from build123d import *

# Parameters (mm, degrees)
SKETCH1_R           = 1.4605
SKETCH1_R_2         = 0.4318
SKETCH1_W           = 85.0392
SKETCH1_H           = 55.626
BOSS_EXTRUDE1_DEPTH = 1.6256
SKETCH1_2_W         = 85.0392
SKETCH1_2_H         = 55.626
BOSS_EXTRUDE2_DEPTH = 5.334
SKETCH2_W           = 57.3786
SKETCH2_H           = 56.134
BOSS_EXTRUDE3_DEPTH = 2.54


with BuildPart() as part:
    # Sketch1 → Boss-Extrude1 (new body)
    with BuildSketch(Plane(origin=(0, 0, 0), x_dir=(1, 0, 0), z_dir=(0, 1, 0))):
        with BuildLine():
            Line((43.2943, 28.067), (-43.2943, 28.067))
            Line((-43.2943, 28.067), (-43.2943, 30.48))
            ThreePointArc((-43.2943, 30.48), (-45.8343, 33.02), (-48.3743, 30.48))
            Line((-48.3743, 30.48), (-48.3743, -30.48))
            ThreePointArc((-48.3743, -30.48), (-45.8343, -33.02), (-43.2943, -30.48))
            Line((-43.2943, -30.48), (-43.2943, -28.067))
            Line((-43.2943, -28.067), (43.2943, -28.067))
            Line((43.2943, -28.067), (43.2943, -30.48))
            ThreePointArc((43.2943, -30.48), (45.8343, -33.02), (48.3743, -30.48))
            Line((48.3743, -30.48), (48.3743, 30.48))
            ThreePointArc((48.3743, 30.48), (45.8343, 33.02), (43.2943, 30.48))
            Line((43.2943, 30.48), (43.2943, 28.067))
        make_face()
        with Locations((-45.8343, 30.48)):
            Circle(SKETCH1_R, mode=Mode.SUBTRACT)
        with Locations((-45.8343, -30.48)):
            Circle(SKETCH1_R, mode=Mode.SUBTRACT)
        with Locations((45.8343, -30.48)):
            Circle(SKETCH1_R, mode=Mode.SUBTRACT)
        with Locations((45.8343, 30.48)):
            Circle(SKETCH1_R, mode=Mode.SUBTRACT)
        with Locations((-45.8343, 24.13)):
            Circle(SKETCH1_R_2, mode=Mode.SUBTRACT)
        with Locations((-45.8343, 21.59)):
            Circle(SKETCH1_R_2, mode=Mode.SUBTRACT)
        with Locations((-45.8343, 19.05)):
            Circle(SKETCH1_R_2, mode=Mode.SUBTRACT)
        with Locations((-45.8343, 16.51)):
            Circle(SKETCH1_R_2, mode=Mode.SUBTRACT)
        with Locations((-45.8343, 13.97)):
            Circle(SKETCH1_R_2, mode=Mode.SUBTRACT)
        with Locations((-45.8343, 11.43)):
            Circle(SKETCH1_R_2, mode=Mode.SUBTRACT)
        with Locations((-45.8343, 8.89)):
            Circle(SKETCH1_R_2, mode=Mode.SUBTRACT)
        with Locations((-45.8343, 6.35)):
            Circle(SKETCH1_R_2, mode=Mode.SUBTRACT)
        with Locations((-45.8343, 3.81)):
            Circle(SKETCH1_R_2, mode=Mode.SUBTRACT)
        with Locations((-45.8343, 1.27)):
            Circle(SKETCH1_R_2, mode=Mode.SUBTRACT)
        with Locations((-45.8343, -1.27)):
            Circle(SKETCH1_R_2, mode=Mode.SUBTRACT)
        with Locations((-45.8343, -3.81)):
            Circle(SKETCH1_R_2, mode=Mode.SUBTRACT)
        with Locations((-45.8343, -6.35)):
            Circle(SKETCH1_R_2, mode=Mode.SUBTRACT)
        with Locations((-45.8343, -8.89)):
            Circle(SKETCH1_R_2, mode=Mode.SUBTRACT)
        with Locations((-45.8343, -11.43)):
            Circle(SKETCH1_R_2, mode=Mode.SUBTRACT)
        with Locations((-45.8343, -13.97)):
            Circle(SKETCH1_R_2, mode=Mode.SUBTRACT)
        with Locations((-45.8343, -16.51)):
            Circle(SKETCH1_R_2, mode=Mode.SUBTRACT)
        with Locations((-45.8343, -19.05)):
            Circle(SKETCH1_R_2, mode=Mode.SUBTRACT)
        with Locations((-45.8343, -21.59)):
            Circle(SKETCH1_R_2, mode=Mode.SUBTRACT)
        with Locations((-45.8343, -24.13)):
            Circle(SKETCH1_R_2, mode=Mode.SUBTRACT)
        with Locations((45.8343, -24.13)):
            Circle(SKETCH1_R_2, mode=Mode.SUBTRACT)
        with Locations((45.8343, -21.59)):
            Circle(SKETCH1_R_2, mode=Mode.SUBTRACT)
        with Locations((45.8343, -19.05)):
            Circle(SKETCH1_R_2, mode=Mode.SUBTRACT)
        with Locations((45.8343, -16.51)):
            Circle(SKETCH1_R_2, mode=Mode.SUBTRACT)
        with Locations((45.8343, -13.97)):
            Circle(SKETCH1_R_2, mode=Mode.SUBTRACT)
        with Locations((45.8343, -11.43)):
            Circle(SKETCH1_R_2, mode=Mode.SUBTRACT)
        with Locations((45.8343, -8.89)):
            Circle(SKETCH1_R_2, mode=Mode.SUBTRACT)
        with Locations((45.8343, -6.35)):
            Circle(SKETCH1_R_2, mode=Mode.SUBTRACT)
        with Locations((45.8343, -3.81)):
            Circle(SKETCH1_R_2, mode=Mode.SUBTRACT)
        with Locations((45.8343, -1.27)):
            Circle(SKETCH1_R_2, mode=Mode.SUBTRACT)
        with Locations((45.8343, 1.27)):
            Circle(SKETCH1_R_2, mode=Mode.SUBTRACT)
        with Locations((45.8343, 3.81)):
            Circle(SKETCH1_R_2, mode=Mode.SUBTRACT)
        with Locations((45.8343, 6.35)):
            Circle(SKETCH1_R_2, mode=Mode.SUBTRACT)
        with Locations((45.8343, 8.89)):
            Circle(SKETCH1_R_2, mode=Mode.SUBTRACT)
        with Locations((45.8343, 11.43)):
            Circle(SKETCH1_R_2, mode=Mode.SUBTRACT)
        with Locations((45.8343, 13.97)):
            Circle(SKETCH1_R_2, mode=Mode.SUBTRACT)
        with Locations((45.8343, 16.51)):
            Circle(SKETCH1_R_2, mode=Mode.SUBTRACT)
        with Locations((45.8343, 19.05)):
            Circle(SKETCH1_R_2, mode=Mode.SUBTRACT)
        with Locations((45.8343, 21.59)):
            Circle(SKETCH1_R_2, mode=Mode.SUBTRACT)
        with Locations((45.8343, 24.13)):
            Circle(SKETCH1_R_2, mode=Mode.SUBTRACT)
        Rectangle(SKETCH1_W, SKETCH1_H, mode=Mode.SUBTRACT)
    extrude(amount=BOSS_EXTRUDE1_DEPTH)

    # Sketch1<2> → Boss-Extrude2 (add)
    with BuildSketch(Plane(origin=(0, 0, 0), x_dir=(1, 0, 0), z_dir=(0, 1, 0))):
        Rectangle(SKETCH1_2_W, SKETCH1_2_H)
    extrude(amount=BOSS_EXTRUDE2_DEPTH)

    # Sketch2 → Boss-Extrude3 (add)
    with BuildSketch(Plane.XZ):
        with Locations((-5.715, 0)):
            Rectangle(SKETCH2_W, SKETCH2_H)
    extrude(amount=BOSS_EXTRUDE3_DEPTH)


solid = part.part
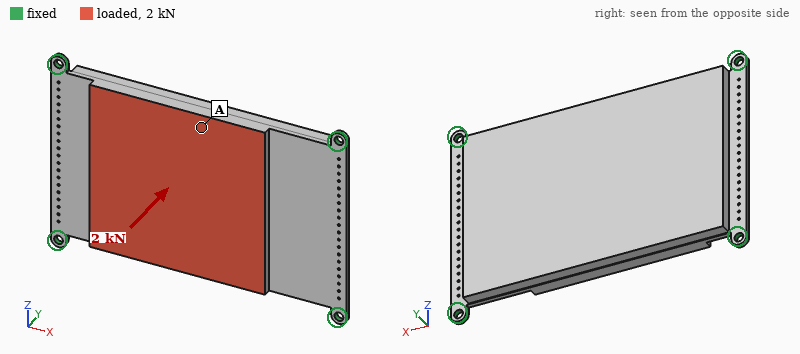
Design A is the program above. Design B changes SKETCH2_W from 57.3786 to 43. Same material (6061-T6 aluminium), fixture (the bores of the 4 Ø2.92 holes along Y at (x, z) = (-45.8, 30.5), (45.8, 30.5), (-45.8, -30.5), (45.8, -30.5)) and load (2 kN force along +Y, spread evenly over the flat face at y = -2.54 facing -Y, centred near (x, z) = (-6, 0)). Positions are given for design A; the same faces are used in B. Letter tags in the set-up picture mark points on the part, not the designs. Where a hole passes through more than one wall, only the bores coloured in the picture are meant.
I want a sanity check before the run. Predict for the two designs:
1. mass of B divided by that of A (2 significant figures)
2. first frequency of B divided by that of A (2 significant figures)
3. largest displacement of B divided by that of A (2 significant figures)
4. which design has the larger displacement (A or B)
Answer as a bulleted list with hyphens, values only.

- 0.94
- 0.97
- 1.2
- B
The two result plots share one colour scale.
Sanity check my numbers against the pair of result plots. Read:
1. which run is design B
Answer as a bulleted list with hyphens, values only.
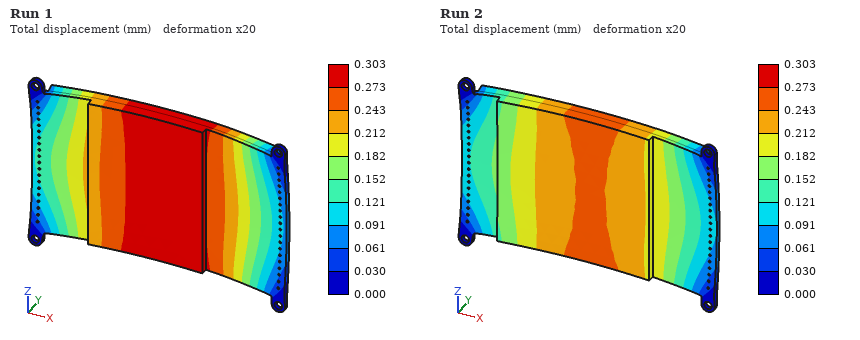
- Run 1
